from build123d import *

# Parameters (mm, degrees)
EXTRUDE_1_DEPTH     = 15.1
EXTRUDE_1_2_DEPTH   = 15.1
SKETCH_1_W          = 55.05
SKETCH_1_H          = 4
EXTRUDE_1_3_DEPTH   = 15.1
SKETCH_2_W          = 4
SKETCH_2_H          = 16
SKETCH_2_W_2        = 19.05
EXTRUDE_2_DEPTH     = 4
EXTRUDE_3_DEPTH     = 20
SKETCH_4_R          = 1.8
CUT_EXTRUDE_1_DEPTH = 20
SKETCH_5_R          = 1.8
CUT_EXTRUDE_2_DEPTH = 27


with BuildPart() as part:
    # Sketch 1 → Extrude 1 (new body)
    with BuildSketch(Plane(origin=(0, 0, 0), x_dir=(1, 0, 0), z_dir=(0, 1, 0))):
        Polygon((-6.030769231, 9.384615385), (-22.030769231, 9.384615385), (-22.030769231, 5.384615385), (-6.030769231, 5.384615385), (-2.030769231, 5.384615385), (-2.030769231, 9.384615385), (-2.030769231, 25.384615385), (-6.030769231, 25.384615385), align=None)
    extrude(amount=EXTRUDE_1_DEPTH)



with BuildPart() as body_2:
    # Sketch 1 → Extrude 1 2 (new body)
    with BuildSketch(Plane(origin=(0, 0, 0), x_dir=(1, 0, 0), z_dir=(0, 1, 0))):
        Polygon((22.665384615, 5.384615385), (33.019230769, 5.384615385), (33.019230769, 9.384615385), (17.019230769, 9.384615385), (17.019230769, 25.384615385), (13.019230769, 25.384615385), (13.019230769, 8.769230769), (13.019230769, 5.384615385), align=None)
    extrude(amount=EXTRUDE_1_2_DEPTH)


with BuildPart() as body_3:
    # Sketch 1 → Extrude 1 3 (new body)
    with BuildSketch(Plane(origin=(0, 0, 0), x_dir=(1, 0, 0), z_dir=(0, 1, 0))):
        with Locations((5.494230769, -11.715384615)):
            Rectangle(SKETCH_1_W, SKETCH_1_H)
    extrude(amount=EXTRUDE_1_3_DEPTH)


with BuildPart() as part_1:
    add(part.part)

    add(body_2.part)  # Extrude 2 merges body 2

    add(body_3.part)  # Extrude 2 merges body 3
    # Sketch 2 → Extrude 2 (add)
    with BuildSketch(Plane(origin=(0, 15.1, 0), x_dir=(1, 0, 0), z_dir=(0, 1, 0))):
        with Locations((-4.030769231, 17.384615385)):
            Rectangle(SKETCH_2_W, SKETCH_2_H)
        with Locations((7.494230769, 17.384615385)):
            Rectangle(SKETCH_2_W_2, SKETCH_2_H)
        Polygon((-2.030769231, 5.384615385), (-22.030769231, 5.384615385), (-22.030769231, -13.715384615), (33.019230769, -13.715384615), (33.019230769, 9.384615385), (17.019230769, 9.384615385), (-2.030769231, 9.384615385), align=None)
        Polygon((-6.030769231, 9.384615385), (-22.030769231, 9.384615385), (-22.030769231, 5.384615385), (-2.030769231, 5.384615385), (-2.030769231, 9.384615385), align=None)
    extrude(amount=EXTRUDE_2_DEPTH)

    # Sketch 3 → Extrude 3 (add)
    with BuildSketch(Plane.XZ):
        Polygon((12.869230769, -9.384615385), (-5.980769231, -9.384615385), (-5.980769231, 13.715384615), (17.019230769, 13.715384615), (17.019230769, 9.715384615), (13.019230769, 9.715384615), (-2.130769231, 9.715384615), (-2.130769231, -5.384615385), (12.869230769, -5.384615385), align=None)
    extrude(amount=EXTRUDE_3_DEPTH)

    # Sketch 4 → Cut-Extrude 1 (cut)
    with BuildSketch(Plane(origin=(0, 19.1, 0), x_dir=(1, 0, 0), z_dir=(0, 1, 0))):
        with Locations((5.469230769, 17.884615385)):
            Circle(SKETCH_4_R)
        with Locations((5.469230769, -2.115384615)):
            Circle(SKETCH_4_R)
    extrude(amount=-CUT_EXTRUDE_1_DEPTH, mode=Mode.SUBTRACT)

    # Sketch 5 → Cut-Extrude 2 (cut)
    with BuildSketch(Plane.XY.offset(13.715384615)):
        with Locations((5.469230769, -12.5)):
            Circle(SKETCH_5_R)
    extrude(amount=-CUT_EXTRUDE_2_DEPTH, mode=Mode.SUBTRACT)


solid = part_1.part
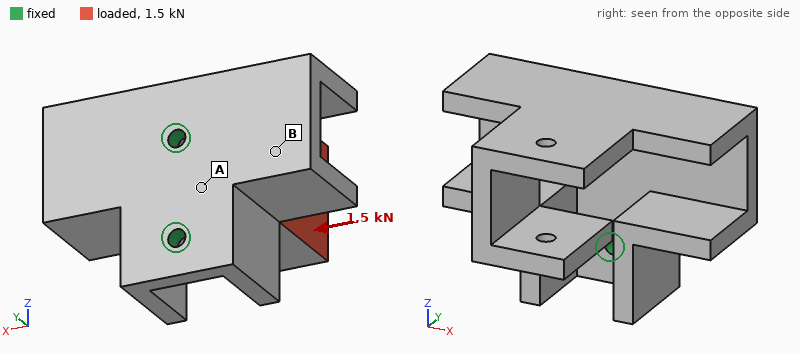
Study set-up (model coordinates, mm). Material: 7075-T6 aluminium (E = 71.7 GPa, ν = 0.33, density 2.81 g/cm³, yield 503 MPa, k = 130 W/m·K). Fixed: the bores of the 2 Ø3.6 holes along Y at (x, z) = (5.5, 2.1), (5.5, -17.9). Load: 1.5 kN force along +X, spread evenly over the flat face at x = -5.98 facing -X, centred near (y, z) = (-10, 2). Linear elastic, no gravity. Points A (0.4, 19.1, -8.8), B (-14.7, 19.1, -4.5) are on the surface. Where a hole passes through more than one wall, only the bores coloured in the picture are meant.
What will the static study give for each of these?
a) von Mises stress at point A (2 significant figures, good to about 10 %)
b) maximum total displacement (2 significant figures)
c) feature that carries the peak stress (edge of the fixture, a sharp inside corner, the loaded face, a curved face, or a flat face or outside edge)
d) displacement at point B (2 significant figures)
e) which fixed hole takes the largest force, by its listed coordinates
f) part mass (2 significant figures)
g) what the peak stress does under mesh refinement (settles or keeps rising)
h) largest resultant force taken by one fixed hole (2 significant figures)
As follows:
150 MPa
0.78 mm
edge of the fixture
0.25 mm
(5.5, 2.1)
52 g
keeps rising
1.4 kN
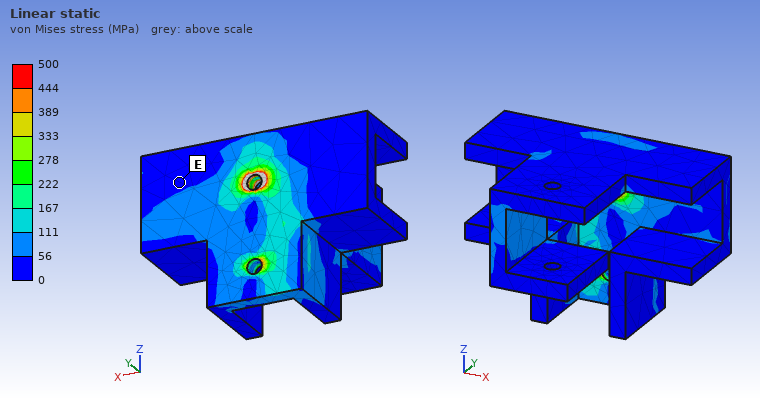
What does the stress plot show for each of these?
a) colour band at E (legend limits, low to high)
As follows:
0 to 56 MPa
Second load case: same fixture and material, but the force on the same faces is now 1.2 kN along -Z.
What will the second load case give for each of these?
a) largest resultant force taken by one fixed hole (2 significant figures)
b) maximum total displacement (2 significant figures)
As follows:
1.5 kN
0.18 mm
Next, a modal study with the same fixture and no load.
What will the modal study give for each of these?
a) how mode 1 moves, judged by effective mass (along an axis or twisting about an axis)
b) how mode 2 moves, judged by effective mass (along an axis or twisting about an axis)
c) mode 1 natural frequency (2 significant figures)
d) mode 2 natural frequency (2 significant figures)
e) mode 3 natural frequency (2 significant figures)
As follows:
along X
along Z
1900 Hz
3300 Hz
5000 Hz
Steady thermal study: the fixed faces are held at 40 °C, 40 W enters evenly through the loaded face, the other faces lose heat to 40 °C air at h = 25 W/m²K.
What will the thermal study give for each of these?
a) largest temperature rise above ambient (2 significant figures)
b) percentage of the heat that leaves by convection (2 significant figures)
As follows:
70 K
15 %
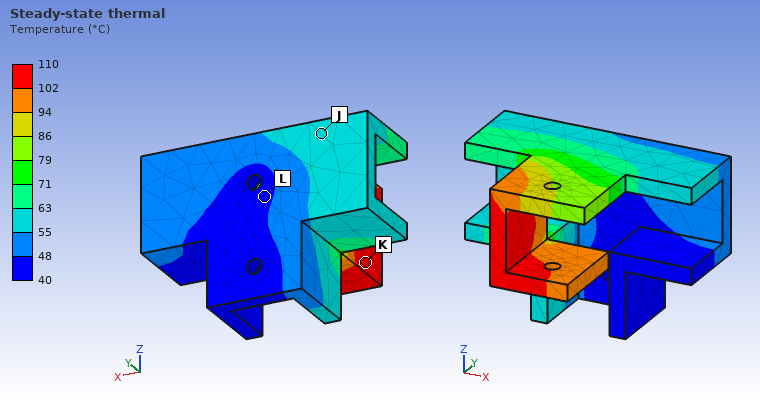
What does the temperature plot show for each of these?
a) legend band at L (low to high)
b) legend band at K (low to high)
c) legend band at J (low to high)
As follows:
40 to 48 °C
102 to 110 °C
55 to 63 °C
